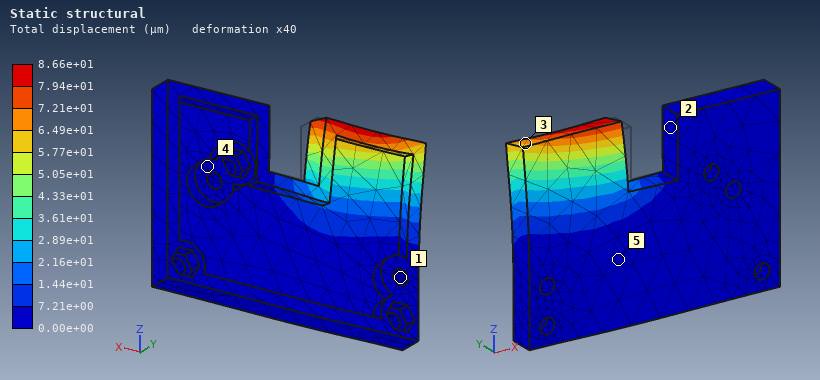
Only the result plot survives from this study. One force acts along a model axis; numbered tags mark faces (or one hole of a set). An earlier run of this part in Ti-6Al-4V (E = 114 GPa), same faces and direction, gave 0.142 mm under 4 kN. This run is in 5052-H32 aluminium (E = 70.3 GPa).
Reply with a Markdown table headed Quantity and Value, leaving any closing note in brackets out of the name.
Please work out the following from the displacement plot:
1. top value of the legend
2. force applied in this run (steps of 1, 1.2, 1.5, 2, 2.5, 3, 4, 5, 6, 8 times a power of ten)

| Quantity | Value |
|---|---|
| top value of the legend | 8.66e+01 µm |
| force applied in this run | 1.5 kN |
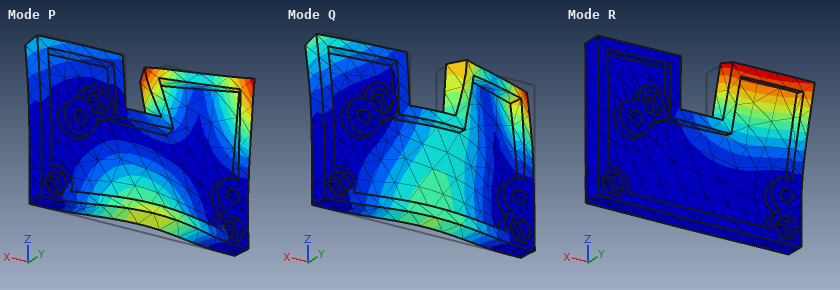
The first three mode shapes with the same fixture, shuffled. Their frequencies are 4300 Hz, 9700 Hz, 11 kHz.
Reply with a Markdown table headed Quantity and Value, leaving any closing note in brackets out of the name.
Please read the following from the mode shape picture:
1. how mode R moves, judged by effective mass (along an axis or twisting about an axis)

| Quantity | Value |
|---|---|
| how mode R moves, judged by effective mass | along Y |
